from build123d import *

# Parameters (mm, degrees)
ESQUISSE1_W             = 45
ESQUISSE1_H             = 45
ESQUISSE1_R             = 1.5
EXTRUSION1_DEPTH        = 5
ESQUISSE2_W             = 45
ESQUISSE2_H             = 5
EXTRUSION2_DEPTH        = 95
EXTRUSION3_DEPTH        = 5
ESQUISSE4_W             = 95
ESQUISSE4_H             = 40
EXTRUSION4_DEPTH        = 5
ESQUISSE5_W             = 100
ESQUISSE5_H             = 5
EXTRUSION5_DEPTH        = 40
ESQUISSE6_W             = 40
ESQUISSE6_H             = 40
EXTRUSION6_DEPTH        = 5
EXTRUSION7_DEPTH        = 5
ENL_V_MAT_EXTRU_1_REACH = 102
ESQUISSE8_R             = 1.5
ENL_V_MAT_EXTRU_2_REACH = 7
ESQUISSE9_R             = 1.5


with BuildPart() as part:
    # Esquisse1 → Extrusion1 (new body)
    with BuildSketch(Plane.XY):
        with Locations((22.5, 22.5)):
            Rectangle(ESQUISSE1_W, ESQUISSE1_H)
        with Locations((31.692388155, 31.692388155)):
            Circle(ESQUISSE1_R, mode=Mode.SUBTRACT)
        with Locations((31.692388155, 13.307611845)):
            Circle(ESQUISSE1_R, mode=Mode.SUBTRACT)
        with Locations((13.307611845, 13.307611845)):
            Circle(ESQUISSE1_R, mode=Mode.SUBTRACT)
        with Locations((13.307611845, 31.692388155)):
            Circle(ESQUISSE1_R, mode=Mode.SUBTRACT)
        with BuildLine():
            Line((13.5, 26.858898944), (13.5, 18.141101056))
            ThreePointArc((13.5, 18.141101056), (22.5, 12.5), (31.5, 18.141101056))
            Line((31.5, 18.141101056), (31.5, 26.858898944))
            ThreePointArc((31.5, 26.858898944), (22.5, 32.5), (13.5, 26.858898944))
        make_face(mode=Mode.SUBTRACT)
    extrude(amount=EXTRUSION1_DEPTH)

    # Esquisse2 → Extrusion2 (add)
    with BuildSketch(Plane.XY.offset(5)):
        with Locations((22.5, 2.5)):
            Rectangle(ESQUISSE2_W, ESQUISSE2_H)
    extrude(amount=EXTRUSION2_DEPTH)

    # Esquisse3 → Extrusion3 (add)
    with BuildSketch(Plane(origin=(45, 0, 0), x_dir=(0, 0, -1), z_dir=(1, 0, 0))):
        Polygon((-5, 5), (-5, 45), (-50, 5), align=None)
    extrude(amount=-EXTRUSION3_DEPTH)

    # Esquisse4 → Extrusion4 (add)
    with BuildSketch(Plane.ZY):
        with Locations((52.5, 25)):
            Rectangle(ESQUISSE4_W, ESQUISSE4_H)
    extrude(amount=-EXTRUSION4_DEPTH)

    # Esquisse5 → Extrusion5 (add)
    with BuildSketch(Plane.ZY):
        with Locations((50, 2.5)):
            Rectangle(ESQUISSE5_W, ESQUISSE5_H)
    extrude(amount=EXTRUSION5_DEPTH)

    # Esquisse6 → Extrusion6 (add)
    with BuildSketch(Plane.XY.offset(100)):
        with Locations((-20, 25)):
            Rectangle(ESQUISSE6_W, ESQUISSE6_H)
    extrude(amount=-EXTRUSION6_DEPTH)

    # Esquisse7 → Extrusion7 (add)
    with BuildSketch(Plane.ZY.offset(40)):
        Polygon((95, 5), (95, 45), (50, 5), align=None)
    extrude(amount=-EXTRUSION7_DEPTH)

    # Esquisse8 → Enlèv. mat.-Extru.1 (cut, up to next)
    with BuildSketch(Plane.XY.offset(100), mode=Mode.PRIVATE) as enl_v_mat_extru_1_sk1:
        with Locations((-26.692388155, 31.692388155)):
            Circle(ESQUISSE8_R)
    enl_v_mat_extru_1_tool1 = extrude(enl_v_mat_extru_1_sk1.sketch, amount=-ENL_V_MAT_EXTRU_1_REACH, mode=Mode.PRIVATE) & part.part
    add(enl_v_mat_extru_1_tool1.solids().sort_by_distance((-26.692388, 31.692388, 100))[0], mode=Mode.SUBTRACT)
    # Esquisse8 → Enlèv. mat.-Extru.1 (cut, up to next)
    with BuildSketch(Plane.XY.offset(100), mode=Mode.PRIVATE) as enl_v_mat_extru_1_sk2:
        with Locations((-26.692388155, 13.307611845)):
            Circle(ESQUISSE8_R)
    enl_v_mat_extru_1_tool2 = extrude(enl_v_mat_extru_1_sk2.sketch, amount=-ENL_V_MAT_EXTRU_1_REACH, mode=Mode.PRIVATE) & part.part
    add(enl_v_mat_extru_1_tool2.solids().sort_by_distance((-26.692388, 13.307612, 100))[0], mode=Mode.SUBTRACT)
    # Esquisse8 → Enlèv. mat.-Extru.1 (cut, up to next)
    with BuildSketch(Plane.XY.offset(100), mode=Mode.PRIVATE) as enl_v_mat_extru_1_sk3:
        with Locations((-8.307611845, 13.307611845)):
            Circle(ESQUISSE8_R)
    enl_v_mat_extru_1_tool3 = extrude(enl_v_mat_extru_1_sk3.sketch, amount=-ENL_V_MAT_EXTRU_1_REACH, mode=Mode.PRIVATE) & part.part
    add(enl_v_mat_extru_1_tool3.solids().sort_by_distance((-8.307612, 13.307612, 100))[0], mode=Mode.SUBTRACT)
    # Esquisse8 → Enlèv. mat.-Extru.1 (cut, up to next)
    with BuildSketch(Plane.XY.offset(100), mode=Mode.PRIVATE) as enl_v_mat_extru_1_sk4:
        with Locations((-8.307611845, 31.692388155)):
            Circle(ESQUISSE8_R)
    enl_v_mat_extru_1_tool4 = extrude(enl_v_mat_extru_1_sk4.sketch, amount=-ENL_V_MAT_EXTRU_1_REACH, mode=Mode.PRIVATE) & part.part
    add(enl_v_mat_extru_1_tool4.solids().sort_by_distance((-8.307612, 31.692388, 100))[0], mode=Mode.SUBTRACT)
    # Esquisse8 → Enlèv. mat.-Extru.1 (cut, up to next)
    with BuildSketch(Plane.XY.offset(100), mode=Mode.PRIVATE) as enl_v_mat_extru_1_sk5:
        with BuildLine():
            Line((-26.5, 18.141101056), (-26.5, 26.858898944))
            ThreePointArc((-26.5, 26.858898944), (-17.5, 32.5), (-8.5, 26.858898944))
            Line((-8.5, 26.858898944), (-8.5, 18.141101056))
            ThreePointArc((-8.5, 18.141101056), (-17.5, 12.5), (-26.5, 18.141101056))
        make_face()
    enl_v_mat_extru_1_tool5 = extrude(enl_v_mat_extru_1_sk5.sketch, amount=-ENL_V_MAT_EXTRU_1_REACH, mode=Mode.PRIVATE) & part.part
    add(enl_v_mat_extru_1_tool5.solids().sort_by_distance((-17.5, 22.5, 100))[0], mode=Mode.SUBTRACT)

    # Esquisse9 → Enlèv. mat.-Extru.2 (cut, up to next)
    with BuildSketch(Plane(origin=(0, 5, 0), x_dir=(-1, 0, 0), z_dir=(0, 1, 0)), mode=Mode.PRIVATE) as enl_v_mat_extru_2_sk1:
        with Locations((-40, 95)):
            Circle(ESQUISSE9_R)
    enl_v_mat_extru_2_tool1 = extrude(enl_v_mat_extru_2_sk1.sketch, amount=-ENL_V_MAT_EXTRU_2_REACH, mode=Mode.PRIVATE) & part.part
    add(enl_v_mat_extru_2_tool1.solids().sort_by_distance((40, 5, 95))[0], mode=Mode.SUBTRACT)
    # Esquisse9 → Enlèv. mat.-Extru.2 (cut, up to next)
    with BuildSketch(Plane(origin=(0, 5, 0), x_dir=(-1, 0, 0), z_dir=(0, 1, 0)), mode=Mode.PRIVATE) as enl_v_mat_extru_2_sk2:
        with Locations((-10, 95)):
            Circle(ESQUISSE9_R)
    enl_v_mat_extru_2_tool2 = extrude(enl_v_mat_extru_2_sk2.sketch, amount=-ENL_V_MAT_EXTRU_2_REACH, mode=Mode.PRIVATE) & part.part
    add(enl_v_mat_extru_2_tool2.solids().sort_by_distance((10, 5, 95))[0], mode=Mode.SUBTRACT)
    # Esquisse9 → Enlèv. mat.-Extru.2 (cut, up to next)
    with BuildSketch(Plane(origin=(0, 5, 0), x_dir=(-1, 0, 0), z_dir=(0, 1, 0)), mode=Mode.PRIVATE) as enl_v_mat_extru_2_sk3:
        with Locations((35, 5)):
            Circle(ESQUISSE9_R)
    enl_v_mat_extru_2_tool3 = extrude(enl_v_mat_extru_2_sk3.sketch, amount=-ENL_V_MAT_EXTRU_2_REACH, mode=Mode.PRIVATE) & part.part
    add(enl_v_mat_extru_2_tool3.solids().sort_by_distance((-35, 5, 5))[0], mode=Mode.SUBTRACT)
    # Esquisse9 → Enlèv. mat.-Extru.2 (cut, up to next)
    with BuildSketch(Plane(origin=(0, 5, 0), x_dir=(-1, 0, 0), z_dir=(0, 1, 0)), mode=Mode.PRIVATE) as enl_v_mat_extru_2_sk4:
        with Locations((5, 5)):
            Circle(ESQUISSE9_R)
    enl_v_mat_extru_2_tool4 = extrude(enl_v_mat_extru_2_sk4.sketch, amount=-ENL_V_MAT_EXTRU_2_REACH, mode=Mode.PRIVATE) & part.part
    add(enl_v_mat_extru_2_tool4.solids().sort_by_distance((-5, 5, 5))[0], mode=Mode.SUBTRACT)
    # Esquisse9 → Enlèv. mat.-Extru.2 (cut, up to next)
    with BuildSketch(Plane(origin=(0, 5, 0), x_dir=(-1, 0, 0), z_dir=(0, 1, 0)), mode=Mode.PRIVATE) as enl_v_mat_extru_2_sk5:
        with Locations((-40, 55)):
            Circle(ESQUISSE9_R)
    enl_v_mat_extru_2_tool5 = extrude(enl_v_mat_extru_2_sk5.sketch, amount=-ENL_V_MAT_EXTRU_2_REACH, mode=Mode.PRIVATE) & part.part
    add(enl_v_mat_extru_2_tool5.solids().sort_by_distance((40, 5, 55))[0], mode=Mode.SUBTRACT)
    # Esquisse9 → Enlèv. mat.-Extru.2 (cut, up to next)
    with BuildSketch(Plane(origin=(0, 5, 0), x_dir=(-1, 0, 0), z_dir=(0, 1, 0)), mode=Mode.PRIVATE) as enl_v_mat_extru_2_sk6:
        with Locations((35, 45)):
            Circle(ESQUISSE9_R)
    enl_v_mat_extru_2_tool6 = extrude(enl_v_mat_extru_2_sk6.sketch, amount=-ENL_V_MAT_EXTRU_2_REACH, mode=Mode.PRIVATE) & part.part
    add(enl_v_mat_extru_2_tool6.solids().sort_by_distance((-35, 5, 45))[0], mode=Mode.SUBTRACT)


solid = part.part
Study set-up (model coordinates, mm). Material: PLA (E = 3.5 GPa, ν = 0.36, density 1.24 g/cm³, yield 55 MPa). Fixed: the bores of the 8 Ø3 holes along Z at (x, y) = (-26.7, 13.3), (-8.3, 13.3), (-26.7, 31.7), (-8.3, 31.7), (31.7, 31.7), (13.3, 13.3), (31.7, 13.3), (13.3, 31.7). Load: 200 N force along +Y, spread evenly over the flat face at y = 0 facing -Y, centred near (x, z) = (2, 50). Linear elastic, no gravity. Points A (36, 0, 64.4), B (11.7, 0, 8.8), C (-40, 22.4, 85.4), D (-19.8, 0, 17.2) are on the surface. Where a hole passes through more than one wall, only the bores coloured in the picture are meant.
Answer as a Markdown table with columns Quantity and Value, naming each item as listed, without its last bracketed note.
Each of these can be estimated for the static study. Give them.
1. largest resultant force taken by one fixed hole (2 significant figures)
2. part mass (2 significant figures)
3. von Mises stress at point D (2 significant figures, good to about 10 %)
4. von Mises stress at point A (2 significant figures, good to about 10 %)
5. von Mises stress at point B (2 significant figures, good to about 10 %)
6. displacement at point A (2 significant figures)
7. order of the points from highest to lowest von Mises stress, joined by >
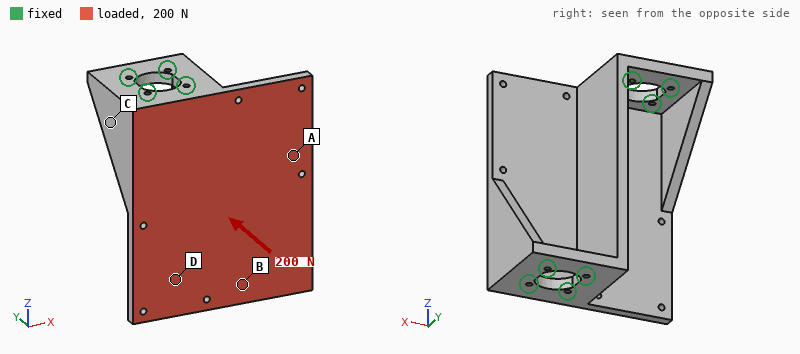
| Quantity | Value |
|---|---|
| largest resultant force taken by one fixed hole | 38 N |
| part mass | 100 g |
| von Mises stress at point D | 1.0 MPa |
| von Mises stress at point A | 1.4 MPa |
| von Mises stress at point B | 0.54 MPa |
| displacement at point A | 0.076 mm |
| order of the points from highest to lowest von Mises stress, joined by > | A > D > B > C |
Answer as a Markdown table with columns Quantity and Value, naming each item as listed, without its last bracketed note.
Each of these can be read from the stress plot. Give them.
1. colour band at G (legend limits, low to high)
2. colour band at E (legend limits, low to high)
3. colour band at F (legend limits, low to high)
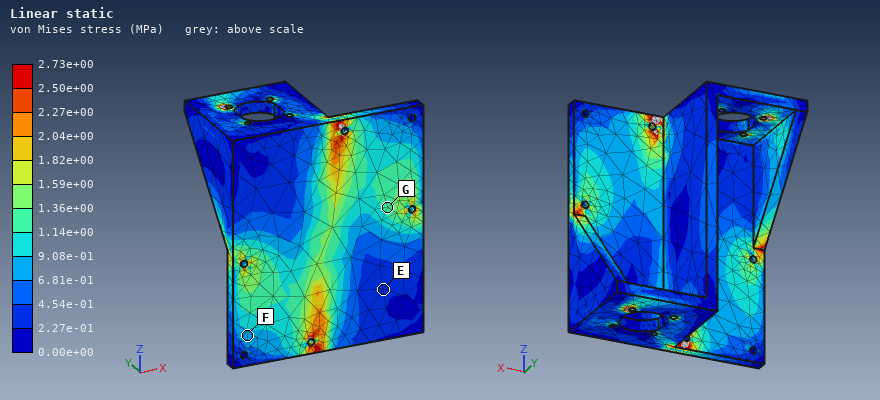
| Quantity | Value |
|---|---|
| colour band at G | 1.14e+00 to 1.36e+00 MPa |
| colour band at E | 2.27e-01 to 4.54e-01 MPa |
| colour band at F | 6.81e-01 to 9.08e-01 MPa |
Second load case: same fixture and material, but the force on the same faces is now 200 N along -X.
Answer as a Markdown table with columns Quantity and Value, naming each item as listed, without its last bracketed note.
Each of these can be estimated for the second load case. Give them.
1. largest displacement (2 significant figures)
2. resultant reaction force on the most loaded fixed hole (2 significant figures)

| Quantity | Value |
|---|---|
| largest displacement | 50 µm |
| resultant reaction force on the most loaded fixed hole | 69 N |
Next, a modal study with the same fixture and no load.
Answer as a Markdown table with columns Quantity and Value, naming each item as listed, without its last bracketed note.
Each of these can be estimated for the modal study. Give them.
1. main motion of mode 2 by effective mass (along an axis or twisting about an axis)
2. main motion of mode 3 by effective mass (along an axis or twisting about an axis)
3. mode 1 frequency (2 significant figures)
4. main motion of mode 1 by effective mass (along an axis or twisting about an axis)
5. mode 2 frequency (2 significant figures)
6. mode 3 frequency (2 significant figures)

| Quantity | Value |
|---|---|
| main motion of mode 2 by effective mass | along Y |
| main motion of mode 3 by effective mass | along X |
| mode 1 frequency | 950 Hz |
| main motion of mode 1 by effective mass | twisting about Z |
| mode 2 frequency | 1000 Hz |
| mode 3 frequency | 1300 Hz |
